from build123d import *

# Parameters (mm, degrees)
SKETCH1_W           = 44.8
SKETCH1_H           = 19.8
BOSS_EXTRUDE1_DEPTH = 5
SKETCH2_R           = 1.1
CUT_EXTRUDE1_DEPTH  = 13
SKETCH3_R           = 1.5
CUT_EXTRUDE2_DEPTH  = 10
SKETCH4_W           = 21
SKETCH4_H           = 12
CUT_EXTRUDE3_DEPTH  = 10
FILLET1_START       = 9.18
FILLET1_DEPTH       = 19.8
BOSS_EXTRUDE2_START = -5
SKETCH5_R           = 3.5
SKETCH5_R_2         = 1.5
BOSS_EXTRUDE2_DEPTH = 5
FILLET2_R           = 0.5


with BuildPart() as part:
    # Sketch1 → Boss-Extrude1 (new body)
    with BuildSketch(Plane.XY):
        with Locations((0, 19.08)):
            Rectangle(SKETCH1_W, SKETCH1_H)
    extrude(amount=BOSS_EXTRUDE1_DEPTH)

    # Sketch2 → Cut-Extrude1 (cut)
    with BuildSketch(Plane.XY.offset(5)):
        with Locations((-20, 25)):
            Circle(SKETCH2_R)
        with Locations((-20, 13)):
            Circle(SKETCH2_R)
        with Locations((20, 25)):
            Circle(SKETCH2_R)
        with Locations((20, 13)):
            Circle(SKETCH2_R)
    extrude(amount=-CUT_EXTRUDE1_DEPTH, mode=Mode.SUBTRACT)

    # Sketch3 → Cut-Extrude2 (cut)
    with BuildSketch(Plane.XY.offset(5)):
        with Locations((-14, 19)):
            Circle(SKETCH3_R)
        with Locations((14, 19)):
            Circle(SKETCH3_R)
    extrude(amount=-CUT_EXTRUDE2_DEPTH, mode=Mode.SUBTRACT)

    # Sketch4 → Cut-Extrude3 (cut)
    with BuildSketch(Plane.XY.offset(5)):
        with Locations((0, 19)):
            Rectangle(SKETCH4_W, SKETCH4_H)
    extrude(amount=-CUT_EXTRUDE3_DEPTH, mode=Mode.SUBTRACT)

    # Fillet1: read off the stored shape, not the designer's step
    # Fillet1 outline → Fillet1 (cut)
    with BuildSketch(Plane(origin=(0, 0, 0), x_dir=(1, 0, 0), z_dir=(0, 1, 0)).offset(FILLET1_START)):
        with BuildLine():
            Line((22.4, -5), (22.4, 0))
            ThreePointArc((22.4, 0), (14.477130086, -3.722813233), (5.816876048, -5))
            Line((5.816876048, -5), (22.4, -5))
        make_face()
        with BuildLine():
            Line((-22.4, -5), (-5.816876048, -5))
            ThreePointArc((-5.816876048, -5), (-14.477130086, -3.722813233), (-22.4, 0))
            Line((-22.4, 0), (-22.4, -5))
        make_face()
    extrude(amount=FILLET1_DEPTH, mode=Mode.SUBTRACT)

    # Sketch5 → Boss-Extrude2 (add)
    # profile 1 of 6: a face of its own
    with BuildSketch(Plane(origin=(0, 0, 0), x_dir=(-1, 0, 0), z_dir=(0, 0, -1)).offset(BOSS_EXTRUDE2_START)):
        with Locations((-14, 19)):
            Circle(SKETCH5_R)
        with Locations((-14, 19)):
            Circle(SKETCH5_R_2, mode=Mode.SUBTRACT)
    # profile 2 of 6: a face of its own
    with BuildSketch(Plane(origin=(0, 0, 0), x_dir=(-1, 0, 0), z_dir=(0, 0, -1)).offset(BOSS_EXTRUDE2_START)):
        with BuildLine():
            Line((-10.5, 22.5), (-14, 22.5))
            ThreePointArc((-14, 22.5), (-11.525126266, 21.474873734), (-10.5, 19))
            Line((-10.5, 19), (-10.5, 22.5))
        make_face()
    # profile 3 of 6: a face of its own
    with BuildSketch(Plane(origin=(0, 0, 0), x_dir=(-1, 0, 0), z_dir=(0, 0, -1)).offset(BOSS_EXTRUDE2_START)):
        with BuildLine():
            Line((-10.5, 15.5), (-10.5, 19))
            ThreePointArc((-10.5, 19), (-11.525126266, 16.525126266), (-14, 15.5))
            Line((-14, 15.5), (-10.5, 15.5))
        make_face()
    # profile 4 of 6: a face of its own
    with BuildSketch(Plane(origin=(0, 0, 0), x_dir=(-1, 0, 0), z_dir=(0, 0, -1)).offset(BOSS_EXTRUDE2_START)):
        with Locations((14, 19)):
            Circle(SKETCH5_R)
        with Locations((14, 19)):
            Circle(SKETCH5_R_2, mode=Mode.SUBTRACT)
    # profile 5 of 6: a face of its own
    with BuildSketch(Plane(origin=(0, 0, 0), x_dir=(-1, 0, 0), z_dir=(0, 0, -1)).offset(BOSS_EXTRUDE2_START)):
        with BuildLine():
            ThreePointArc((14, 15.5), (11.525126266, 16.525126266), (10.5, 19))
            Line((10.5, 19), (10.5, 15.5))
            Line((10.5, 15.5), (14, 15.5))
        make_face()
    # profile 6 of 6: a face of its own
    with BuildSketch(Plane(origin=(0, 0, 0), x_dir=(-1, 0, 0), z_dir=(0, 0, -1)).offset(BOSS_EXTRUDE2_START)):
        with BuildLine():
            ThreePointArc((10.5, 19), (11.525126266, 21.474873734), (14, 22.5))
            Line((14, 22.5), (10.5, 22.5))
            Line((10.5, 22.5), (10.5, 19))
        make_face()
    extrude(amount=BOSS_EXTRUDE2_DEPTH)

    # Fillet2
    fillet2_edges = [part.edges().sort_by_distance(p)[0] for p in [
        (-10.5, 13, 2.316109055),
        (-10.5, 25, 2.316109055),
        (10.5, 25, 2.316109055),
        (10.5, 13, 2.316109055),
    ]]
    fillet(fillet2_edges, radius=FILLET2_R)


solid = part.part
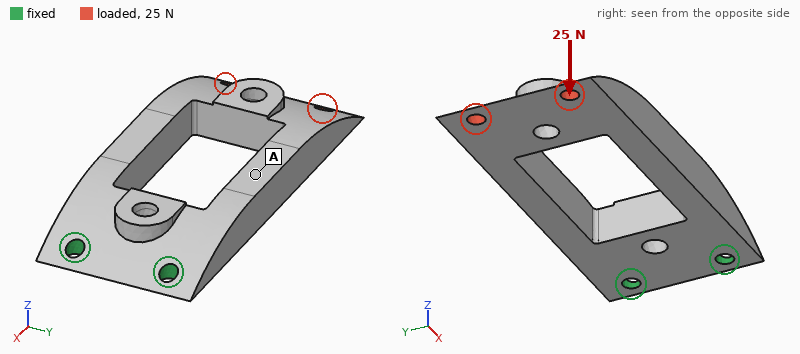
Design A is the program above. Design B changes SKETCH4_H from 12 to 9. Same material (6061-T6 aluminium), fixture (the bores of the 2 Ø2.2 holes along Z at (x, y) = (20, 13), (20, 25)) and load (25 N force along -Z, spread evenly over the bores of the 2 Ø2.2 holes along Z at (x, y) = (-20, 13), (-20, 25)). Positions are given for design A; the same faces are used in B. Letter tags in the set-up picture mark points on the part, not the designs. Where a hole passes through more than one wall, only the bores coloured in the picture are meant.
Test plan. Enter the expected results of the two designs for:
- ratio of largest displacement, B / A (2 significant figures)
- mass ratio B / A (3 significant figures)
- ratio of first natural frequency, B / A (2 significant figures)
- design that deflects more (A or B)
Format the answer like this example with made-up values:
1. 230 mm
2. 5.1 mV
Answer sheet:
1. 0.91
2. 1.15
3. 0.98
4. A
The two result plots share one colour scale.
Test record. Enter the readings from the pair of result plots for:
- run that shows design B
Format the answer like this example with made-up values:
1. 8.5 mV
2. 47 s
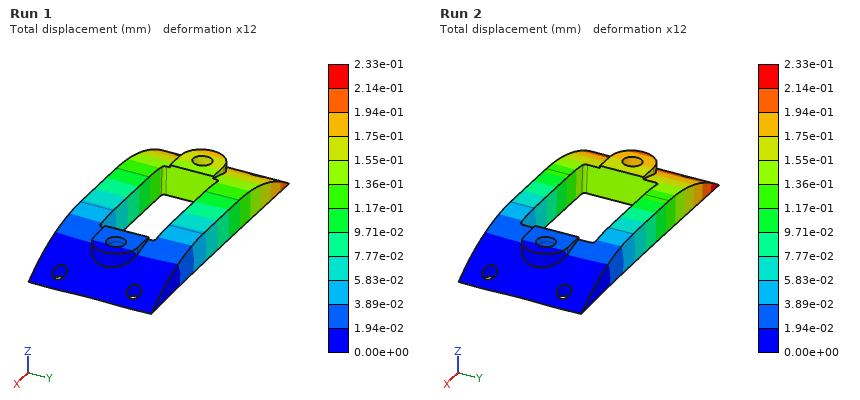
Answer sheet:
1. Run 1
